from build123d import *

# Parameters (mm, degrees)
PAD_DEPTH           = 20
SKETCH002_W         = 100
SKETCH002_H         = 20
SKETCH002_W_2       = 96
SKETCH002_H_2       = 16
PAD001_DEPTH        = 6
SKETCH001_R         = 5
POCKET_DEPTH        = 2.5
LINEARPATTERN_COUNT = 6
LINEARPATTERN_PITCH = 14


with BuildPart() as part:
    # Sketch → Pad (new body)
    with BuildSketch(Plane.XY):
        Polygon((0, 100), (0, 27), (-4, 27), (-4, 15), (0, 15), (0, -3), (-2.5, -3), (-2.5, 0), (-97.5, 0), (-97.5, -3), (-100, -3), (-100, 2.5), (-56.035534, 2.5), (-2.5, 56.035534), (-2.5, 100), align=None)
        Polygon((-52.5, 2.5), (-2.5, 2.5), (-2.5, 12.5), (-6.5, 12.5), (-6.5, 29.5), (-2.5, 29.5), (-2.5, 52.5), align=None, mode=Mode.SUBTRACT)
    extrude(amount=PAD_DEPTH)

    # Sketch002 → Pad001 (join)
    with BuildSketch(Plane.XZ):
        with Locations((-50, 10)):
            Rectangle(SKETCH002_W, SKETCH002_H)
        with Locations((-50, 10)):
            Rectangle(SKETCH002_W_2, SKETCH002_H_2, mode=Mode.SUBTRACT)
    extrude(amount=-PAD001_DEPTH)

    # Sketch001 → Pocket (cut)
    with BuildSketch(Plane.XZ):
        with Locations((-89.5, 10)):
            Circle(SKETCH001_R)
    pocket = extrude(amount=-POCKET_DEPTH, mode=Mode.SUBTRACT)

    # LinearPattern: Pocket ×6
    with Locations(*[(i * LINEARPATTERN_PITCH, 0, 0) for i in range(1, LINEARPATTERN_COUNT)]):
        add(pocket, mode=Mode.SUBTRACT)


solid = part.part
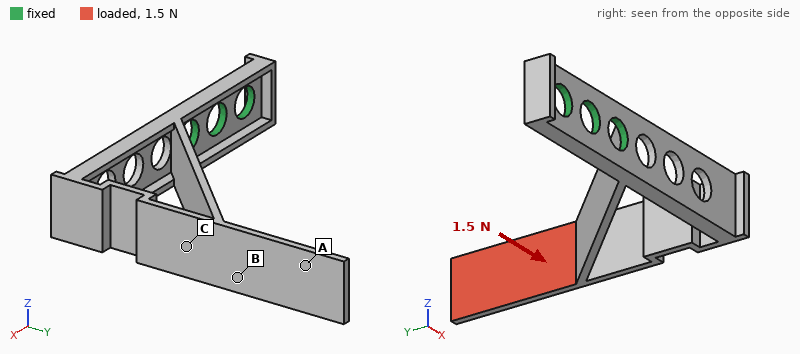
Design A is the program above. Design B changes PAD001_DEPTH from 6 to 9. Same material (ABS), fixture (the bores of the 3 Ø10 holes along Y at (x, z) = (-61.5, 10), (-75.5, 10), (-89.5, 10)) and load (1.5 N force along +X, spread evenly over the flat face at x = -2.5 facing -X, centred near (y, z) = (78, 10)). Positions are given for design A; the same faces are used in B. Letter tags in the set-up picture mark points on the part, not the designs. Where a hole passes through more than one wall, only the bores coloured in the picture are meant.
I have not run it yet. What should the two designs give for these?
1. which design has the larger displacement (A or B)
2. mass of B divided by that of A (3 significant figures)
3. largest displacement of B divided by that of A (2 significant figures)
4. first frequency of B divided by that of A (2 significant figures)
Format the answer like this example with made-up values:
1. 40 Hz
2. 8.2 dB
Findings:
1. A
2. 1.08
3. 0.59
4. 1.5
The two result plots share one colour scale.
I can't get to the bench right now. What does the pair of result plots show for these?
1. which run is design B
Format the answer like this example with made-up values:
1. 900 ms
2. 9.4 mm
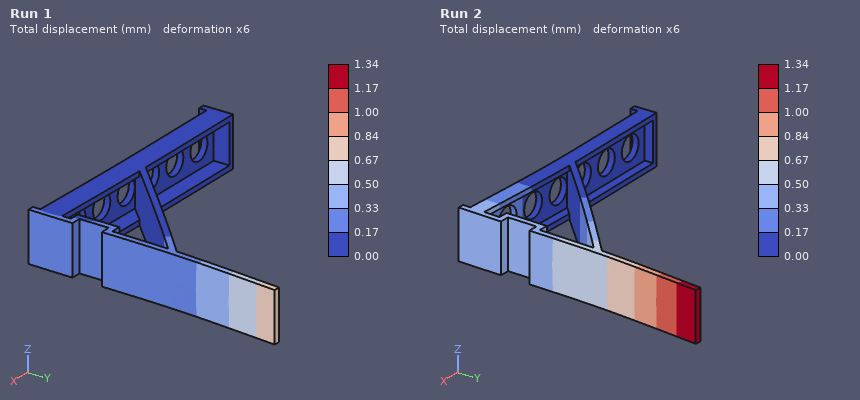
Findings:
1. Run 1
